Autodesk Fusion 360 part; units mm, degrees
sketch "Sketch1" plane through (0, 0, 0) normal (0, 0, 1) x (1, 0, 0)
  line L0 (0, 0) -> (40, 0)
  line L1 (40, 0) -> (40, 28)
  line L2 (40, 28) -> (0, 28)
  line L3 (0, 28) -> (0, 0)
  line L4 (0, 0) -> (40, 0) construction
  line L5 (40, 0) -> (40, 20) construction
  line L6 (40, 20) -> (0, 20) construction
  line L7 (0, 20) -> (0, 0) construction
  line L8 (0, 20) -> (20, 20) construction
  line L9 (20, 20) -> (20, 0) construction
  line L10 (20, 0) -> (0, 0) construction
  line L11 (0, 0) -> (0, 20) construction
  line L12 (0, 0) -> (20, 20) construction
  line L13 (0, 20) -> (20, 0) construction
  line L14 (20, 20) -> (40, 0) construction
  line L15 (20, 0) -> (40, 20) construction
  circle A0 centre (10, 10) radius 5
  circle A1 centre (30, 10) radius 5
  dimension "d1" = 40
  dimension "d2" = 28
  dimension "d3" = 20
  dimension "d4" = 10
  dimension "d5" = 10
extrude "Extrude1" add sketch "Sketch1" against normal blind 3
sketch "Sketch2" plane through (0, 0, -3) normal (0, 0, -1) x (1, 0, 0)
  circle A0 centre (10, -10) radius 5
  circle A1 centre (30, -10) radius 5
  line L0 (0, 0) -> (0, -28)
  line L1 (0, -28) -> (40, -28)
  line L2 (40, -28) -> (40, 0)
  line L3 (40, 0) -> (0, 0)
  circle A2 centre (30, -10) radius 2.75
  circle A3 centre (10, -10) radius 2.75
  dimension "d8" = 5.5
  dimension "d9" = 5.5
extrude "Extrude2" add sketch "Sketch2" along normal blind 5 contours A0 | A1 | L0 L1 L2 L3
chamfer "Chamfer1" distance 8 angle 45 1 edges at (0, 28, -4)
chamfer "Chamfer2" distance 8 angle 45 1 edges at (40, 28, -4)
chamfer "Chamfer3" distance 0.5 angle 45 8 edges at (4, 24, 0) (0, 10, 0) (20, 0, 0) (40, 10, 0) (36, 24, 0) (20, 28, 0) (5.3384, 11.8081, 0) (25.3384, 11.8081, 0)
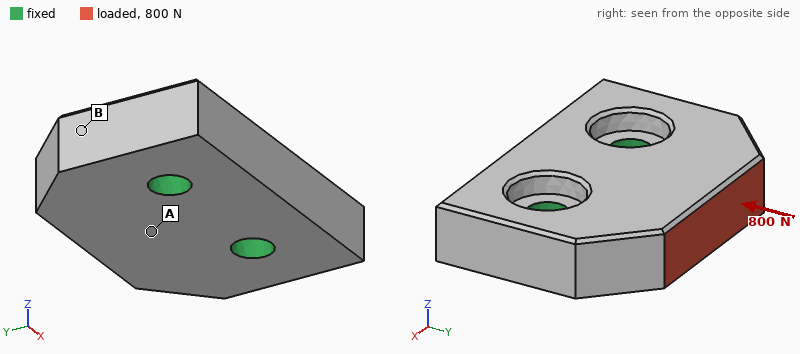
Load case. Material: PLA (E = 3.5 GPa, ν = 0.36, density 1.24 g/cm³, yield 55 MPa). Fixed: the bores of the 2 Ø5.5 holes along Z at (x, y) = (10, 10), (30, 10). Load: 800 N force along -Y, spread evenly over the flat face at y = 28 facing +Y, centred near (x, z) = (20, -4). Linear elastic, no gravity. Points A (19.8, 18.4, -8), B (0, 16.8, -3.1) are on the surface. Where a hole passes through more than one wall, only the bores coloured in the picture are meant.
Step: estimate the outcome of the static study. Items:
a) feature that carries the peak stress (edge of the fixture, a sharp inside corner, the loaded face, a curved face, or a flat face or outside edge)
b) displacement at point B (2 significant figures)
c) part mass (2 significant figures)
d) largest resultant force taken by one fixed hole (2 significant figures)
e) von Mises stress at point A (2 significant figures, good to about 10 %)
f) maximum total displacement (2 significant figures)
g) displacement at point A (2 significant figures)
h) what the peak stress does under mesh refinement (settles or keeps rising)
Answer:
edge of the fixture
13 µm
9.6 g
410 N
3.3 MPa
41 µm
15 µm
keeps rising
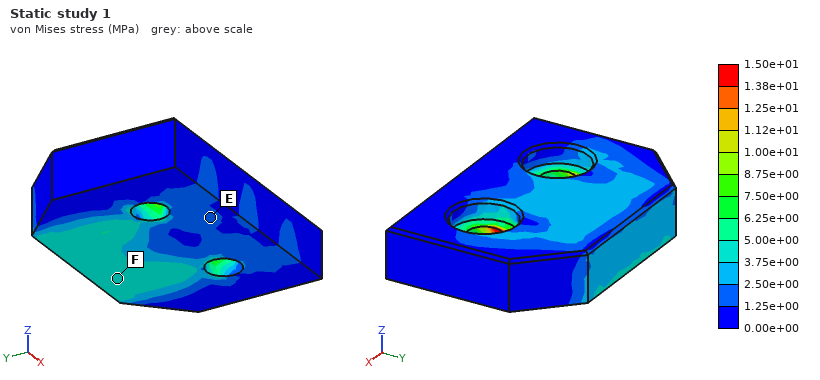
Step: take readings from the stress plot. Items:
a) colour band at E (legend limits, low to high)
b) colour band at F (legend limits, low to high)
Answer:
1.25e+00 to 2.50e+00 MPa
3.75e+00 to 5.00e+00 MPa
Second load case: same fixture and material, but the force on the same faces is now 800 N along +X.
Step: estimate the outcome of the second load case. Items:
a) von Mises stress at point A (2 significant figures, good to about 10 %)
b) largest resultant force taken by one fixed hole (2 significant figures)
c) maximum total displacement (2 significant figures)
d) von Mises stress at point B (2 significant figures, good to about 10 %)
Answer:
9.3 MPa
710 N
79 µm
2.4 MPa
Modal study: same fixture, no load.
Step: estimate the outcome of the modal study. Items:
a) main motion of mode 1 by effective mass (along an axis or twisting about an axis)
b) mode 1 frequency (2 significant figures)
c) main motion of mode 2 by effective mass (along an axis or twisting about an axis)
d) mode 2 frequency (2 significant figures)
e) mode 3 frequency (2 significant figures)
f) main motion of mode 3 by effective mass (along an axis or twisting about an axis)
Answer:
along Z
4700 Hz
twisting about Y
7800 Hz
10 kHz
along X
